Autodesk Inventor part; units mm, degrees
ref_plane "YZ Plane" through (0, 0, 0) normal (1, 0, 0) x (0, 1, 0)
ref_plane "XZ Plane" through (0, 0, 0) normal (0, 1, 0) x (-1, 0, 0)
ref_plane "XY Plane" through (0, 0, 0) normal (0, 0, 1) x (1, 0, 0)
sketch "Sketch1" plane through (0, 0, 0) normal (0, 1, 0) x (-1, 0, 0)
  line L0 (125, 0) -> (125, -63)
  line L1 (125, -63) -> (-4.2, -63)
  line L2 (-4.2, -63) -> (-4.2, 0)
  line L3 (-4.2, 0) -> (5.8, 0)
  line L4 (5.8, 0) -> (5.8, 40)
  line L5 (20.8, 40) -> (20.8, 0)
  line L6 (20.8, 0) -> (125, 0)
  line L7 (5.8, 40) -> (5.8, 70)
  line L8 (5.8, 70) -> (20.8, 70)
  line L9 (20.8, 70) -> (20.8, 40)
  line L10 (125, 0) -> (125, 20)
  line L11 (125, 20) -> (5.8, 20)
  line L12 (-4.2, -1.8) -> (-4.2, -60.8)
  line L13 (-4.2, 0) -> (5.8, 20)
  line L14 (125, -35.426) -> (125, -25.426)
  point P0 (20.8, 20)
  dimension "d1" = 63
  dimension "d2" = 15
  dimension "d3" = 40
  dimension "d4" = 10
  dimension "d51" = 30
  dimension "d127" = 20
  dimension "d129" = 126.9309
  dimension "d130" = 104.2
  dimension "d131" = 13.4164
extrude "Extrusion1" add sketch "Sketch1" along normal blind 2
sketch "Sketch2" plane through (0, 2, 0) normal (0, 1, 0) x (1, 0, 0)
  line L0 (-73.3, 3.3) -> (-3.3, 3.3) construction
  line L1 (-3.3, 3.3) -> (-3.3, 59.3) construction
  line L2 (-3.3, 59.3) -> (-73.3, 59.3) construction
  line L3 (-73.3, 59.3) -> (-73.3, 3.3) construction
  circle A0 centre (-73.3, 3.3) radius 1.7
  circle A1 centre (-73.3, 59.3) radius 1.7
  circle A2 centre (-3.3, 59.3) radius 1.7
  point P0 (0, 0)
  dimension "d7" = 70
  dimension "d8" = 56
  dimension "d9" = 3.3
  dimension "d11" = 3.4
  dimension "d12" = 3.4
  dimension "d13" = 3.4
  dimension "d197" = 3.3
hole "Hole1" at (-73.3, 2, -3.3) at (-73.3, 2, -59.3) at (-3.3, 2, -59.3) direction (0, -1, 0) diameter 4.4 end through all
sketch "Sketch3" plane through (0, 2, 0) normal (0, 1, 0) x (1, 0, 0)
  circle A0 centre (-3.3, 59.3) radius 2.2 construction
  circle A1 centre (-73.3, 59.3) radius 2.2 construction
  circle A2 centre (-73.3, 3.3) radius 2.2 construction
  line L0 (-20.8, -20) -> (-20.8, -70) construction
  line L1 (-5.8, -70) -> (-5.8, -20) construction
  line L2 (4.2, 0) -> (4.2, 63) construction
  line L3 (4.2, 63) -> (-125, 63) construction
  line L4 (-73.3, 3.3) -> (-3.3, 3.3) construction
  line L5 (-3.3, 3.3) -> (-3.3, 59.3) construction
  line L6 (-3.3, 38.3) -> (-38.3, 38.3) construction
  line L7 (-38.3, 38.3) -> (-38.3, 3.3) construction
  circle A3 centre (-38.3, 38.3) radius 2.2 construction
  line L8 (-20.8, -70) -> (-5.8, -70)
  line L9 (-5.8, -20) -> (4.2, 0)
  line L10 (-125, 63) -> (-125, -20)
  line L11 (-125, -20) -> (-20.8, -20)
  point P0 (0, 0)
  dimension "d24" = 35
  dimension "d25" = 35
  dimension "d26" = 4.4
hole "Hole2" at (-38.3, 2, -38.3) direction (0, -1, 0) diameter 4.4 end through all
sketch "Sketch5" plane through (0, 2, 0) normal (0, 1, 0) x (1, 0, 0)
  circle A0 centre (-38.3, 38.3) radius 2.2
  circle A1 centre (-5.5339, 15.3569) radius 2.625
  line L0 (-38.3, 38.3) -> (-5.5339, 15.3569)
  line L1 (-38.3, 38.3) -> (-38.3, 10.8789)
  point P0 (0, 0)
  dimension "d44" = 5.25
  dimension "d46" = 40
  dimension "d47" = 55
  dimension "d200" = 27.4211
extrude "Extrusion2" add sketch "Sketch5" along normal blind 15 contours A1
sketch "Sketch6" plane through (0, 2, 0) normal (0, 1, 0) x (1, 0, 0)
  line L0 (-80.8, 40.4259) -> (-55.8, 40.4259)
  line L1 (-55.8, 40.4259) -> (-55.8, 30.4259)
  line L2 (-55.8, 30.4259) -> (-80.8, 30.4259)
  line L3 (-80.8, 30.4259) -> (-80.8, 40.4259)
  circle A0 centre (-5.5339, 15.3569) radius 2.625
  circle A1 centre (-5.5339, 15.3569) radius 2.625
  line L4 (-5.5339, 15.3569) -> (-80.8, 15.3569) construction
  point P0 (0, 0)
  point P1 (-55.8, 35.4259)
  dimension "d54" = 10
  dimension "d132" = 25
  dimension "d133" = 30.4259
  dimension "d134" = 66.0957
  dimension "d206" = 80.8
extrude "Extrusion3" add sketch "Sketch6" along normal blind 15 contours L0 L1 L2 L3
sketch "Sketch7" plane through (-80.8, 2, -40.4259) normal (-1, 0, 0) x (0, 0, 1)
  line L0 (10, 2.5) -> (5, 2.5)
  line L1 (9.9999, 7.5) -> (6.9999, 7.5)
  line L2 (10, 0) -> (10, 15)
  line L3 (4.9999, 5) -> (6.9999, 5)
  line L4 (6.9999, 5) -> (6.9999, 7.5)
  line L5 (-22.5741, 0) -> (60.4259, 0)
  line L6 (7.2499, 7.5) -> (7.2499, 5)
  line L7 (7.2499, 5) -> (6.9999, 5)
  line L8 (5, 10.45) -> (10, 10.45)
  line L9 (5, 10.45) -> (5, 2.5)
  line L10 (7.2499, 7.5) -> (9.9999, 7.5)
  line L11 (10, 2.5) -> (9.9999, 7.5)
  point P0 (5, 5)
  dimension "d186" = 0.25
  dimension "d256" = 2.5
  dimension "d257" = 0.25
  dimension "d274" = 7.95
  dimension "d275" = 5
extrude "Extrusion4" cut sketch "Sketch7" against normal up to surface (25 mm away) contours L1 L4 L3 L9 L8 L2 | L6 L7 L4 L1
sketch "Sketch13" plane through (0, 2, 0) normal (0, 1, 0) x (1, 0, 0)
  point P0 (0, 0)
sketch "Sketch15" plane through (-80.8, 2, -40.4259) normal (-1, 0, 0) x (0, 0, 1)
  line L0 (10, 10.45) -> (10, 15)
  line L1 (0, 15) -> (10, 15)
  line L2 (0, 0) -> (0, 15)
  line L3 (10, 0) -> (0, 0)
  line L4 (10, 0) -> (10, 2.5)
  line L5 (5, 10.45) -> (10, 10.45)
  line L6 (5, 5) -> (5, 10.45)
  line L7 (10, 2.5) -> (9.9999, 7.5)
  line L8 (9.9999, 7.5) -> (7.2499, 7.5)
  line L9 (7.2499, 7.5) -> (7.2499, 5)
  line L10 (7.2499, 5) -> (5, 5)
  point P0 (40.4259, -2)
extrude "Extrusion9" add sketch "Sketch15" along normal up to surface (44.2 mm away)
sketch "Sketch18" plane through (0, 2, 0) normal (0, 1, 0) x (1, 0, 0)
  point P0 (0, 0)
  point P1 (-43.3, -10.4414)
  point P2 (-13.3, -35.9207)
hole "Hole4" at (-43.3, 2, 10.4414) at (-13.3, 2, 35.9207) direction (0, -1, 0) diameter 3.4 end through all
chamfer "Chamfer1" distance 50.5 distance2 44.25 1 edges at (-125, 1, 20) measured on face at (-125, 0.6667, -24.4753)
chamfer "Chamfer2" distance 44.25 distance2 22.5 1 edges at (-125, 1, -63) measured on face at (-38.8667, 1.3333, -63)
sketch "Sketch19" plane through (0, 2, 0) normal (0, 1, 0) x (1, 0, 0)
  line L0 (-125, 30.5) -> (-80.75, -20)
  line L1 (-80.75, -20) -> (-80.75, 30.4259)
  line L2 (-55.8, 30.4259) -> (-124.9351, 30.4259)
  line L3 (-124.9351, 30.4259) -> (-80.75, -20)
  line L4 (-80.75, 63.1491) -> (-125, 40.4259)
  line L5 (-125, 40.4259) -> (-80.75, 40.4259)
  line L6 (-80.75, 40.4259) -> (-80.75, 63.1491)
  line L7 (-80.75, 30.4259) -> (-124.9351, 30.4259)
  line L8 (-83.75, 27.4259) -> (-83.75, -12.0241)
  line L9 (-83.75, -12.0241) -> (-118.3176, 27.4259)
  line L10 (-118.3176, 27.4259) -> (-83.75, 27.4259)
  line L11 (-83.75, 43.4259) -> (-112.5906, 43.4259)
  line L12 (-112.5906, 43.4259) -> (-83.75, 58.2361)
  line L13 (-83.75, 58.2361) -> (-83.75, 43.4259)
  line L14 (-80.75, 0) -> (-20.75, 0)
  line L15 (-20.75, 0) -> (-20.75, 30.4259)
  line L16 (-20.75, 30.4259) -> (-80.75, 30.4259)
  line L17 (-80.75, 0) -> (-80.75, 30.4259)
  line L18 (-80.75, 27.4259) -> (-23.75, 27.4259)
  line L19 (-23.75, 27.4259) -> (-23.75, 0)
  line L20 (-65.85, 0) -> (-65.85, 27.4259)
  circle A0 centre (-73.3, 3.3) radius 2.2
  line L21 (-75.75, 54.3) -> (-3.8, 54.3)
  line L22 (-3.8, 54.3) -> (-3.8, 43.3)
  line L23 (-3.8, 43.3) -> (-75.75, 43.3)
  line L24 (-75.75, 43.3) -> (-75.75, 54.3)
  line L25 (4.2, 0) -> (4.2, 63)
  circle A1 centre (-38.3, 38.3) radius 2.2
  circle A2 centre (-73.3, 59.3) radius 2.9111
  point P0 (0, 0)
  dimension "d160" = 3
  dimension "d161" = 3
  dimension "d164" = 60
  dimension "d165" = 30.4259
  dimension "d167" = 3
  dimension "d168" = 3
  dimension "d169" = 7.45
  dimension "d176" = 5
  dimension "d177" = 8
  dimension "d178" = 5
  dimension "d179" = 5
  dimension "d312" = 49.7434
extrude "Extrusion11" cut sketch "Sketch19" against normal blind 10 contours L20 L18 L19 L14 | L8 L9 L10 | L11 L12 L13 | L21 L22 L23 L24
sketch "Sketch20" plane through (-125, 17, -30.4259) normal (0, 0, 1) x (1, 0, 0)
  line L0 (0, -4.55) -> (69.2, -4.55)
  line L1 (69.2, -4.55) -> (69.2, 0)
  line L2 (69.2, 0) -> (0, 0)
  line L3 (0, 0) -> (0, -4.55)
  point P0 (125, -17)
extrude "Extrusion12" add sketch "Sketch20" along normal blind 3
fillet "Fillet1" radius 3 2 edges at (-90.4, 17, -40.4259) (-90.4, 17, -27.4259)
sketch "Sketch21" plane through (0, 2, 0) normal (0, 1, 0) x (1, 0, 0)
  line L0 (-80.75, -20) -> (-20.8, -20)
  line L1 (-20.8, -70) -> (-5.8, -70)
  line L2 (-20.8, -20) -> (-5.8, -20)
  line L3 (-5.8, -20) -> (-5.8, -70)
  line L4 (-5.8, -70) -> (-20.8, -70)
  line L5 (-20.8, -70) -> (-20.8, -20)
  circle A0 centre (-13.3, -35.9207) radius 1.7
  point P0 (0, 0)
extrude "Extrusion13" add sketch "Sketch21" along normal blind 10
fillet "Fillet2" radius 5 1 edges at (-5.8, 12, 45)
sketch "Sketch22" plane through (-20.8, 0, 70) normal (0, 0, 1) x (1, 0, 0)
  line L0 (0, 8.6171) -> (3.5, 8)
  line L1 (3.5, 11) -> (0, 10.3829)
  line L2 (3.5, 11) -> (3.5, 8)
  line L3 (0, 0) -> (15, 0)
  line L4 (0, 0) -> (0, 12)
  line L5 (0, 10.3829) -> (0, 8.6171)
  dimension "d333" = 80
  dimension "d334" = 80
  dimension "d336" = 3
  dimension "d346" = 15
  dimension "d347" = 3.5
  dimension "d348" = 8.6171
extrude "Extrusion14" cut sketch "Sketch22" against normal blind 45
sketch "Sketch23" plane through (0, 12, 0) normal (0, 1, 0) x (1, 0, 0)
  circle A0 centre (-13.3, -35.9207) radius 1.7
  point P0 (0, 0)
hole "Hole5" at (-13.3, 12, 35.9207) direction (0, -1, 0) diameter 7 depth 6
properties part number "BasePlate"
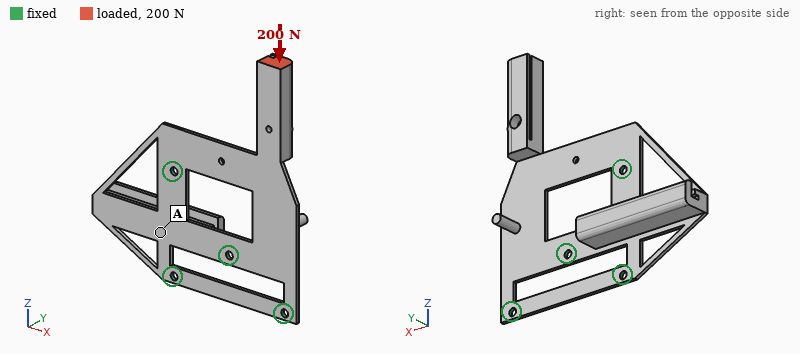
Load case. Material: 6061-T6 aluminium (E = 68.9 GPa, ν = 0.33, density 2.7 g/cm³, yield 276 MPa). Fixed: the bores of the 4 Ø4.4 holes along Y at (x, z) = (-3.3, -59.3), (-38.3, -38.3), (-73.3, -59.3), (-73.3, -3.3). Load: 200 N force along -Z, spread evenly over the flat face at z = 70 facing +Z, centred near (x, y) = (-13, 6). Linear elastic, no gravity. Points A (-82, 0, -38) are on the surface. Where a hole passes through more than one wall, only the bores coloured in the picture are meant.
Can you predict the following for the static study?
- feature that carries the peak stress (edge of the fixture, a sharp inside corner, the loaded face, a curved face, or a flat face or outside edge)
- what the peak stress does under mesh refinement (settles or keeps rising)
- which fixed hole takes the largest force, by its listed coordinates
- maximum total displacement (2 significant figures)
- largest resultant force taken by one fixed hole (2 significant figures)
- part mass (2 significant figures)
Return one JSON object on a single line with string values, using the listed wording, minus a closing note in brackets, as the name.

{"feature that carries the peak stress": "a sharp inside corner", "what the peak stress does under mesh refinement": "keeps rising", "which fixed hole takes the largest force, by its listed coordinates": "(-3.3, -59.3)", "maximum total displacement": "2.0 mm", "largest resultant force taken by one fixed hole": "120 N", "part mass": "82 g"}
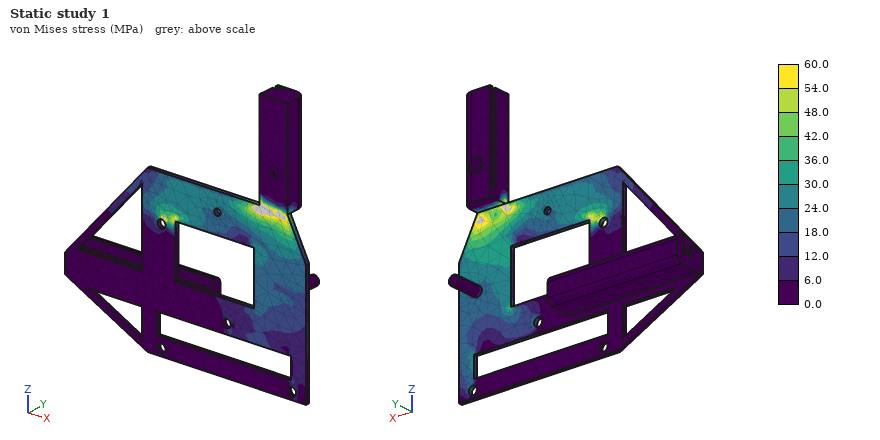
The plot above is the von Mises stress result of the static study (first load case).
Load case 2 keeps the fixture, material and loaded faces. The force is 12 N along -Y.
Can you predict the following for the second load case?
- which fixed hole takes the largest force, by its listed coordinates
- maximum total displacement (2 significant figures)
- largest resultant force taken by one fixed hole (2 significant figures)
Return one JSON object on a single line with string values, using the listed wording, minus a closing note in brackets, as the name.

{"which fixed hole takes the largest force, by its listed coordinates": "(-73.3, -3.3)", "maximum total displacement": "2.2 mm", "largest resultant force taken by one fixed hole": "10 N"}
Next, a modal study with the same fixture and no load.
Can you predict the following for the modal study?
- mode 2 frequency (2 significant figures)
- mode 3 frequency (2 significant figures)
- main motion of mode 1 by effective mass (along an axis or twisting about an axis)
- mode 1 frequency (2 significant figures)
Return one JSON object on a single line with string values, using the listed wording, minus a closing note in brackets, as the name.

{"mode 2 frequency": "590 Hz", "mode 3 frequency": "590 Hz", "main motion of mode 1 by effective mass": "along Y", "mode 1 frequency": "110 Hz"}
